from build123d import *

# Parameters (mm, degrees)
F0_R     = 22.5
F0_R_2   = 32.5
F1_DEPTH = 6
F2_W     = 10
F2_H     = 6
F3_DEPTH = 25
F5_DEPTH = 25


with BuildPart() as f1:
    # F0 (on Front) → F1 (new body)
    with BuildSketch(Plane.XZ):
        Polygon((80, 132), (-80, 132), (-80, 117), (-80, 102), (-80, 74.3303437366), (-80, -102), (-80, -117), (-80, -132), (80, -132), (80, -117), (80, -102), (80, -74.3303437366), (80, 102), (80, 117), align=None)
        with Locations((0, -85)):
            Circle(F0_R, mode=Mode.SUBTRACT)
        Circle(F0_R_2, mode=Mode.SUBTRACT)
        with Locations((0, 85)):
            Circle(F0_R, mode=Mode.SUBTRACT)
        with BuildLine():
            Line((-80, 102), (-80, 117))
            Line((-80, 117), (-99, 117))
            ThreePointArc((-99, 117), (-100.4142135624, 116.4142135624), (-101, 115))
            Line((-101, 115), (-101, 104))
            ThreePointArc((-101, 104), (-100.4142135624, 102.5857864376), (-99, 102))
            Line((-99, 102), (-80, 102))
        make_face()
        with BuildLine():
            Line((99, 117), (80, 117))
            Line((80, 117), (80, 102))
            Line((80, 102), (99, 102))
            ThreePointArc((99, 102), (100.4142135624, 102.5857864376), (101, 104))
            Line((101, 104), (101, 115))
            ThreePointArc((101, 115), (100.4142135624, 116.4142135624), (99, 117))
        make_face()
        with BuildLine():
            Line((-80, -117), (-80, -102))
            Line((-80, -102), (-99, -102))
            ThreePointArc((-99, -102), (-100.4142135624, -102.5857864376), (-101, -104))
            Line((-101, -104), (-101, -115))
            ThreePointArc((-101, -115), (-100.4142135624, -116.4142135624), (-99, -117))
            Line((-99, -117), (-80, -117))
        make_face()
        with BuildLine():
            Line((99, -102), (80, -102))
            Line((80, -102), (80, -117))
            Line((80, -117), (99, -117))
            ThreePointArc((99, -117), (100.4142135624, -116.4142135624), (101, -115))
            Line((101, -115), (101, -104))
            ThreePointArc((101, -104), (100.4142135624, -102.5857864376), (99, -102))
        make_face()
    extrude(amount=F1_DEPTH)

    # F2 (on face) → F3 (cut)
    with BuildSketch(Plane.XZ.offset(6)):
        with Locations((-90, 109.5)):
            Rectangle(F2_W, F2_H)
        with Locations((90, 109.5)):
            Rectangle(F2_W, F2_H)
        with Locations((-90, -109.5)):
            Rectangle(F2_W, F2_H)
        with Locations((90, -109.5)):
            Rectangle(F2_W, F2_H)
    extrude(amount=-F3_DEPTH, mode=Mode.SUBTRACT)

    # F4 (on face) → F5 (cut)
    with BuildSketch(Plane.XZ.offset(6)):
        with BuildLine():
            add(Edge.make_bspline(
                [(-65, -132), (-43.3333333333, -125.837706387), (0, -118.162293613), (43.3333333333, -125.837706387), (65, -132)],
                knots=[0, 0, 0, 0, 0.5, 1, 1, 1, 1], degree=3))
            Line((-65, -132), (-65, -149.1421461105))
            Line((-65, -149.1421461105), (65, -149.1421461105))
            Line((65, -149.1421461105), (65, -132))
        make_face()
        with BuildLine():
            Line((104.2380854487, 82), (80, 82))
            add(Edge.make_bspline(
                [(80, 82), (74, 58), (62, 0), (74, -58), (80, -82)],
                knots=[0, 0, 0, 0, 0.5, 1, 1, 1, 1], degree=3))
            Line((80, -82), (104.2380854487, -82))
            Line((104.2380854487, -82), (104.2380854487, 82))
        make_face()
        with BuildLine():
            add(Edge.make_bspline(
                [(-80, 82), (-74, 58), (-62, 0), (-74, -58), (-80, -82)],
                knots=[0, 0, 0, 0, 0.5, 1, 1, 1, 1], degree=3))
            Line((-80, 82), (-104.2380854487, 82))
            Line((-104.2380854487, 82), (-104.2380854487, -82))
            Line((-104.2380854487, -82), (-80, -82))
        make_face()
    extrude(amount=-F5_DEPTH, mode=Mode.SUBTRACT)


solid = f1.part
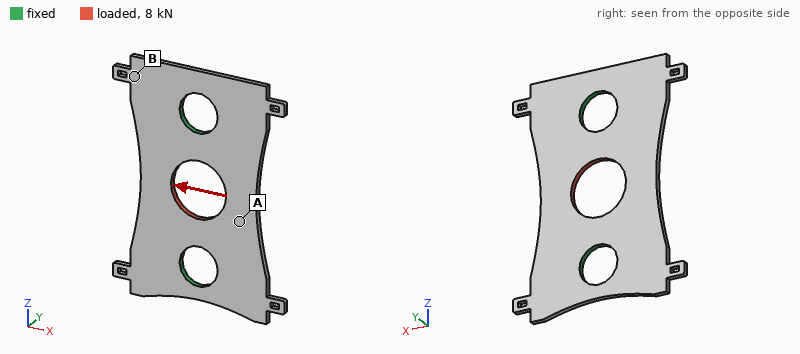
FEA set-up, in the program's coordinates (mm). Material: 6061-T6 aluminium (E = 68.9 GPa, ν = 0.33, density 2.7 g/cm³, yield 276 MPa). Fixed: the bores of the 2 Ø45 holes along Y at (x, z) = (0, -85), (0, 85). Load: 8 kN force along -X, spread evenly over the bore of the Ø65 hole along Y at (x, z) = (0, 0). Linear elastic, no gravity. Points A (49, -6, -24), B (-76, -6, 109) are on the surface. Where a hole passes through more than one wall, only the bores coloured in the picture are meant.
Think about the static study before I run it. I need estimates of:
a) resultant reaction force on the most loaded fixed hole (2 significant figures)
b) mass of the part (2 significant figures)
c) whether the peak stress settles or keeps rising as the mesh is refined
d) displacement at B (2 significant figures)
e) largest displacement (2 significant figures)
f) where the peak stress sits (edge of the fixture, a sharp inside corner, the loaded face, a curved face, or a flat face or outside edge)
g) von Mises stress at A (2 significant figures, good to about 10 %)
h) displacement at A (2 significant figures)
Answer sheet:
4.0 kN
540 g
keeps rising
5.5 µm
17 µm
edge of the fixture
8.4 MPa
13 µm
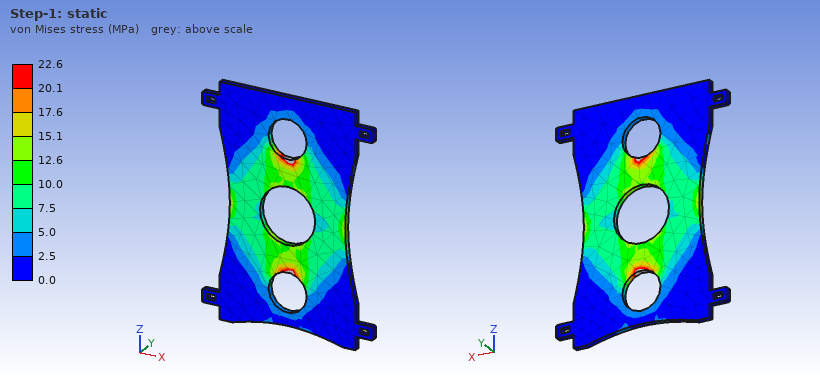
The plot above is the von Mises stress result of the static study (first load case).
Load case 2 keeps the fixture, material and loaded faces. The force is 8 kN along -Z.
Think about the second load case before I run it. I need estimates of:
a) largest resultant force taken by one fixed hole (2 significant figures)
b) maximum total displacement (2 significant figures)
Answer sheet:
4.0 kN
8.3 µm
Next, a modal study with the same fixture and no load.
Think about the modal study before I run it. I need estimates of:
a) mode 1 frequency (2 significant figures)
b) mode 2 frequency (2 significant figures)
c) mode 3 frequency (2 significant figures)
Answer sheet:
1100 Hz
1100 Hz
1200 Hz
